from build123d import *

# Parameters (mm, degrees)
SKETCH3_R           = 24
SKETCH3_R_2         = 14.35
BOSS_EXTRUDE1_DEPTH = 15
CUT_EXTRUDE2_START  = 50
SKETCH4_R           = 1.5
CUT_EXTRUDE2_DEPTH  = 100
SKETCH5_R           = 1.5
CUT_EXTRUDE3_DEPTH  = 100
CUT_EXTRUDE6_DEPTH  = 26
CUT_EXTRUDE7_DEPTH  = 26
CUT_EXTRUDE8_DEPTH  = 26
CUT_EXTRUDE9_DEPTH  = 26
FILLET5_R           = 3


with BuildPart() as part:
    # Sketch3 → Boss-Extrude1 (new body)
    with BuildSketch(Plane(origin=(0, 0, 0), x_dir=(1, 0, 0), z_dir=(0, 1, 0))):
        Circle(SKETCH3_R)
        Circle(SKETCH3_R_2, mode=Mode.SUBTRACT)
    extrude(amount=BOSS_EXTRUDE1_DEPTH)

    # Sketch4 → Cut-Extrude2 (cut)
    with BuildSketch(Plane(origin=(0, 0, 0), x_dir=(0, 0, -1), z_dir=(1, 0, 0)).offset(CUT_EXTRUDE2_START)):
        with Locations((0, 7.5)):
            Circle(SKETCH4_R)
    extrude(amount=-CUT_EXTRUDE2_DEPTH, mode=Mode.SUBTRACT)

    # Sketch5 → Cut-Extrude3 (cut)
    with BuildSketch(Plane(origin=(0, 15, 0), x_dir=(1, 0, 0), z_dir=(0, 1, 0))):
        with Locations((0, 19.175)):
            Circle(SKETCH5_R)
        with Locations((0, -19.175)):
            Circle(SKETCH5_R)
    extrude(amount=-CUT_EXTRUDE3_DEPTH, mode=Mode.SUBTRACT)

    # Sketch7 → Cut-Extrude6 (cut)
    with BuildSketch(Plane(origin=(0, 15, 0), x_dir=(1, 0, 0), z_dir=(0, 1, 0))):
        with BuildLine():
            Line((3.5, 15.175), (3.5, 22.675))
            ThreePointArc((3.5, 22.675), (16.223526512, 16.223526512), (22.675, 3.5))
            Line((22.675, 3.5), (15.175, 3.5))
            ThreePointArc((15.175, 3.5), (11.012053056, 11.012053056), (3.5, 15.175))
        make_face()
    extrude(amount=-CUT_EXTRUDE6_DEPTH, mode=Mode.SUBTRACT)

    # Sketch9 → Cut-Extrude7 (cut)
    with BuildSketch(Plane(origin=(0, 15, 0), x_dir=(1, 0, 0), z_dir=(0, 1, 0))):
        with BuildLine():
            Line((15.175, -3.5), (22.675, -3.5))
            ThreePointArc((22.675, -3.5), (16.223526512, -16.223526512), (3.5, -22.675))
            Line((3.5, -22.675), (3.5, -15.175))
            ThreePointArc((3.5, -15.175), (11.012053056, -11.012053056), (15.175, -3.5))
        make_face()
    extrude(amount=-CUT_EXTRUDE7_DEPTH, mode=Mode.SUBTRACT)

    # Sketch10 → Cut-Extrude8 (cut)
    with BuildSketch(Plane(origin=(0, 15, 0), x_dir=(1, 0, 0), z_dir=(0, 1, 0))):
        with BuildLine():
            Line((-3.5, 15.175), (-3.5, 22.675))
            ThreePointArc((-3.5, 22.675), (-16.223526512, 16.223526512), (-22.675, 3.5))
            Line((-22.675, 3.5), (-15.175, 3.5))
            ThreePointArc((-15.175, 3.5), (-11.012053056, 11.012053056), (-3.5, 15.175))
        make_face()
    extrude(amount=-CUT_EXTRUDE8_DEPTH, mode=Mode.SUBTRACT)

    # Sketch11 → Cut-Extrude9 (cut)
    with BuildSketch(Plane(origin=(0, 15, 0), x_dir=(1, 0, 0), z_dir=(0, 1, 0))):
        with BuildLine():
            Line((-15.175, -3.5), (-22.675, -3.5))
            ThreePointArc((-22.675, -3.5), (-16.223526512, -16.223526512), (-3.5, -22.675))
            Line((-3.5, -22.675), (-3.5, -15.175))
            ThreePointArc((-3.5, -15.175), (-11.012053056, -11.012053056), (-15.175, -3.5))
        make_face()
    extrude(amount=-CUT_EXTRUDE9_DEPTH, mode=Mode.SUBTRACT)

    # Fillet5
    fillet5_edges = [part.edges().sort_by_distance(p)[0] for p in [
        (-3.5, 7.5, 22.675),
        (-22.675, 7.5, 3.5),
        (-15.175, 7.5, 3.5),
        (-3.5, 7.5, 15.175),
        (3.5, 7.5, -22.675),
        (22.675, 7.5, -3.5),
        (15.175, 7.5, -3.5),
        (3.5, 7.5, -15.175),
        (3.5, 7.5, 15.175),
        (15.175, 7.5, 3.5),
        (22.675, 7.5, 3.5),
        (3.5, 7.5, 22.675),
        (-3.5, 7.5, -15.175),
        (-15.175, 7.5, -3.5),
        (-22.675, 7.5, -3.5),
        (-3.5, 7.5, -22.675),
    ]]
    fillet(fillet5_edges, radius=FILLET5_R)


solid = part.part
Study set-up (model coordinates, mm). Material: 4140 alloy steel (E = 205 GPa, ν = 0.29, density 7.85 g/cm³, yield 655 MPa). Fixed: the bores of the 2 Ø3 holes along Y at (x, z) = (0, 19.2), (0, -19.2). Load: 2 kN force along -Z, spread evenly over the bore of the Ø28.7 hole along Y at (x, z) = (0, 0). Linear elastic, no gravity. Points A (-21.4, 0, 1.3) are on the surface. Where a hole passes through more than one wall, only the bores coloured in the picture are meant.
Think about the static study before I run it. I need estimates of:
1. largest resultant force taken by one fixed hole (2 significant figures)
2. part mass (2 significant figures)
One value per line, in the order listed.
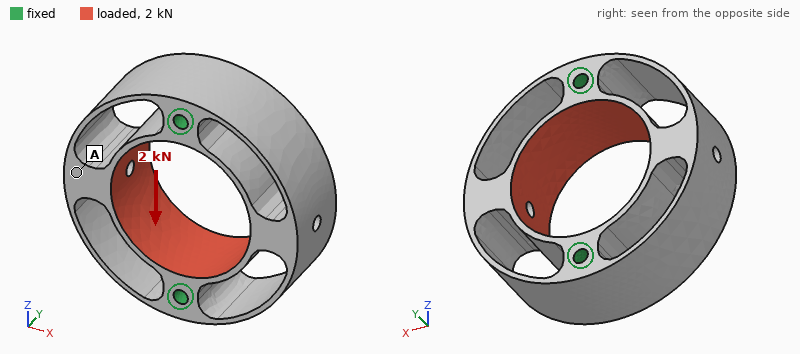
1.0 kN
58 g
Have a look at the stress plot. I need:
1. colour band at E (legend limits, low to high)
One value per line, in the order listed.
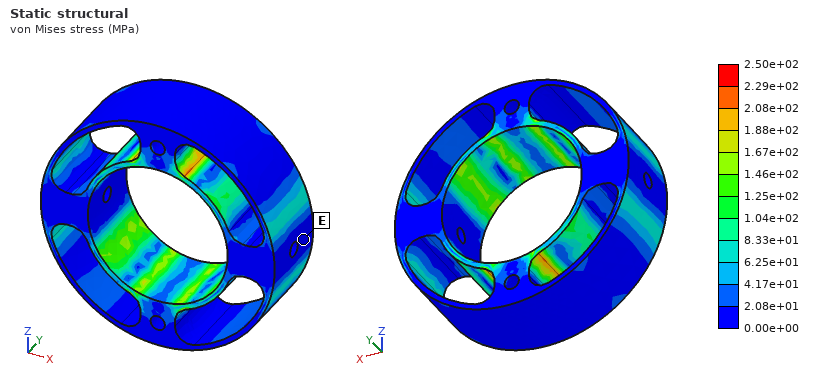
0.00e+00 to 2.08e+01 MPa
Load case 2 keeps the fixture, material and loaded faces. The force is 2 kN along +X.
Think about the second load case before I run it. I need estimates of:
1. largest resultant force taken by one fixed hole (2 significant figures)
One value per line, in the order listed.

1.0 kN
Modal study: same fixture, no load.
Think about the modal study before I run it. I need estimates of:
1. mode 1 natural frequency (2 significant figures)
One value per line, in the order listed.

6800 Hz
